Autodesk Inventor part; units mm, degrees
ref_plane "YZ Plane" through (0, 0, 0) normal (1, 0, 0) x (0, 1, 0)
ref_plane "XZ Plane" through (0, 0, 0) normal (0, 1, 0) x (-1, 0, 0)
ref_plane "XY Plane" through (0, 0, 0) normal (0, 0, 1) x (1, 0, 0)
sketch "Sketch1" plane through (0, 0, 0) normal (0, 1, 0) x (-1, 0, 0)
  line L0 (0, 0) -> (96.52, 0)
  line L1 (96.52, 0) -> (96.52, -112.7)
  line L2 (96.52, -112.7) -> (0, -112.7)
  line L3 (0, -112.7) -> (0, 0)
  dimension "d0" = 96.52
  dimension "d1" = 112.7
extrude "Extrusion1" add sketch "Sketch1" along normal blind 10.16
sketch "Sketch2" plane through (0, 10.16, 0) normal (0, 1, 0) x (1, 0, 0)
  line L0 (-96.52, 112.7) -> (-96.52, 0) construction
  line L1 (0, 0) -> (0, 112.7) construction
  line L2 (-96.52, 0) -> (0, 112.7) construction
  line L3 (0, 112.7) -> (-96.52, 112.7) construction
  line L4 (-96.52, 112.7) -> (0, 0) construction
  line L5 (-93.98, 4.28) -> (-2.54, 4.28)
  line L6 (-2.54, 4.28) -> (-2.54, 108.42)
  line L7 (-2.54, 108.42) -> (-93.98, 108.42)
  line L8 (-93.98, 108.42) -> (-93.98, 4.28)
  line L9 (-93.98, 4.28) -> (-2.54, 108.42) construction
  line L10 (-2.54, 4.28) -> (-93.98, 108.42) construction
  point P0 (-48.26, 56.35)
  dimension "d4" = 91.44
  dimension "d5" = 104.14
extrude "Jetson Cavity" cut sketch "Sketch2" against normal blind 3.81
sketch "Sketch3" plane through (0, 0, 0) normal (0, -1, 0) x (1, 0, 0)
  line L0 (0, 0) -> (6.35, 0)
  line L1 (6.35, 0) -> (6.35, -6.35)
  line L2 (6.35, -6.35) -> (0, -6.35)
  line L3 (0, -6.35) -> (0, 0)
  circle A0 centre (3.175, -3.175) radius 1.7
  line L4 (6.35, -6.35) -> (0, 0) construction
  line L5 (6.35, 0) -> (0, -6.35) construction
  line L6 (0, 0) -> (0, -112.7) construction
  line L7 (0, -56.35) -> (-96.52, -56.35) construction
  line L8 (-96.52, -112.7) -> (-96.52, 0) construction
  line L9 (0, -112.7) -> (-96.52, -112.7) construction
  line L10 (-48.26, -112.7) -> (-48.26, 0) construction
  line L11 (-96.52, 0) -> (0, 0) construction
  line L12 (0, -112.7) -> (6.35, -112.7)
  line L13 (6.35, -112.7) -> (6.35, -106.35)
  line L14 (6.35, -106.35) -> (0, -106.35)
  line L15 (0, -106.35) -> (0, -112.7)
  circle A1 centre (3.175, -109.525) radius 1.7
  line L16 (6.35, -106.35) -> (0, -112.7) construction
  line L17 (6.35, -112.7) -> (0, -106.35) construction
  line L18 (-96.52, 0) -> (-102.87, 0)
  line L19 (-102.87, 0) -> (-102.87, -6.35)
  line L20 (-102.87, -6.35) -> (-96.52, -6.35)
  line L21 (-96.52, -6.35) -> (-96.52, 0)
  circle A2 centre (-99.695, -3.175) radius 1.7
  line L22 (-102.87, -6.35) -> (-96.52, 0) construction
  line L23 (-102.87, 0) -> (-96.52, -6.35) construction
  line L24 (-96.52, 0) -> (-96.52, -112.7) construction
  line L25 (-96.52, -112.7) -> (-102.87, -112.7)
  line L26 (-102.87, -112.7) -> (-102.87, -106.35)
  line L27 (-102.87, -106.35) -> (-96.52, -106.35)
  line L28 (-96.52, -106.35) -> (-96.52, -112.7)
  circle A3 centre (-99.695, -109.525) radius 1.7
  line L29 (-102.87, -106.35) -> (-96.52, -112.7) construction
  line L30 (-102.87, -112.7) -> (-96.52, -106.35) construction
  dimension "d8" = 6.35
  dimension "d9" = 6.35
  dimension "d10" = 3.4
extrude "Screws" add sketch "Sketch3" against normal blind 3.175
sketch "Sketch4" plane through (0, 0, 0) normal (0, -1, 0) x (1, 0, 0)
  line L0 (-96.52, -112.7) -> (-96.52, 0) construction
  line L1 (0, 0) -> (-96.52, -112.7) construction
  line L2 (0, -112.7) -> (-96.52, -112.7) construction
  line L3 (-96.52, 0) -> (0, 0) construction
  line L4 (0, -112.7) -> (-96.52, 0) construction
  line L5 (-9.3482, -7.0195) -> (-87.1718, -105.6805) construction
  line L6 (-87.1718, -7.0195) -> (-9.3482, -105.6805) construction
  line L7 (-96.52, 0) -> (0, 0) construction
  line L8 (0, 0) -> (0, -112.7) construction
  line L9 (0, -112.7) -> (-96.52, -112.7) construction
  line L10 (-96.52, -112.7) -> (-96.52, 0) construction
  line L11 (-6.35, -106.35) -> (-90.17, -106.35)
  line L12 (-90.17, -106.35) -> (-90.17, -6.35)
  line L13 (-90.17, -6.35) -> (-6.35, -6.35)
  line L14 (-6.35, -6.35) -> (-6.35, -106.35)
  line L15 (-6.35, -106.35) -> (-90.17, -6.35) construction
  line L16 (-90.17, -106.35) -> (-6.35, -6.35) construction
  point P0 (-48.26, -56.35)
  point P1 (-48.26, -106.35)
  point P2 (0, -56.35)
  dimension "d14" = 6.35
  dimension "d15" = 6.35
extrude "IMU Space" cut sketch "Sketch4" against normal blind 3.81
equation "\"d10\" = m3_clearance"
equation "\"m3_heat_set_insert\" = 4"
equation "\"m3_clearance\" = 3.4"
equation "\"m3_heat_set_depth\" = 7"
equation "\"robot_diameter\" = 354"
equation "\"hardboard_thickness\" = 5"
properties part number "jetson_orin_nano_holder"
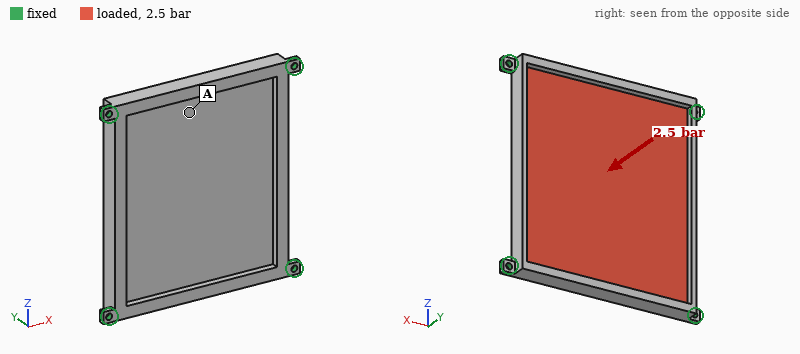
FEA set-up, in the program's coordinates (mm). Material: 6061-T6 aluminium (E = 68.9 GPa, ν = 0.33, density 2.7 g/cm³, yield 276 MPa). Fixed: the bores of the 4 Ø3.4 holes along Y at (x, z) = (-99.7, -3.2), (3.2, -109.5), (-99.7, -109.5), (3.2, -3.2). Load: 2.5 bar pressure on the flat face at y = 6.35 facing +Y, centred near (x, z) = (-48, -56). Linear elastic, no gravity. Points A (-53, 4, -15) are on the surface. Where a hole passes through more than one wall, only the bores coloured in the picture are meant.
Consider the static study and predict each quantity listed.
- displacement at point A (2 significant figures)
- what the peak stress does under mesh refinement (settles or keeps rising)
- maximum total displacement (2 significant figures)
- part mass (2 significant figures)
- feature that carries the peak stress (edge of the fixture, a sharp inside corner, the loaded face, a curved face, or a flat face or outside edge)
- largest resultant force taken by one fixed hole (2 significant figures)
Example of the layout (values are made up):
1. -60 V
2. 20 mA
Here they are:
1. 0.33 mm
2. keeps rising
3. 0.75 mm
4. 120 g
5. edge of the fixture
6. 2.3 kN
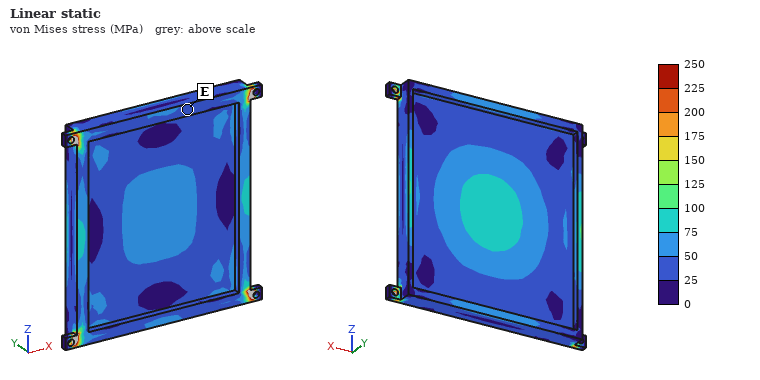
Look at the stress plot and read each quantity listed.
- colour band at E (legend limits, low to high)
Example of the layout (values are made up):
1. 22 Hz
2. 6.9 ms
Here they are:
1. 25 to 50 MPa
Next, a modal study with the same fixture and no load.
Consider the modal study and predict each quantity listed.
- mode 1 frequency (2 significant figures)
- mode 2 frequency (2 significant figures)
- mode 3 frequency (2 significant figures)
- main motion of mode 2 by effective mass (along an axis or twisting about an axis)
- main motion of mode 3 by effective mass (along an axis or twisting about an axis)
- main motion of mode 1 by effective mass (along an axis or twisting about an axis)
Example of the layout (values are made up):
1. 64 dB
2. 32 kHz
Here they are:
1. 1300 Hz
2. 2200 Hz
3. 2500 Hz
4. twisting about Z
5. twisting about X
6. along Y
